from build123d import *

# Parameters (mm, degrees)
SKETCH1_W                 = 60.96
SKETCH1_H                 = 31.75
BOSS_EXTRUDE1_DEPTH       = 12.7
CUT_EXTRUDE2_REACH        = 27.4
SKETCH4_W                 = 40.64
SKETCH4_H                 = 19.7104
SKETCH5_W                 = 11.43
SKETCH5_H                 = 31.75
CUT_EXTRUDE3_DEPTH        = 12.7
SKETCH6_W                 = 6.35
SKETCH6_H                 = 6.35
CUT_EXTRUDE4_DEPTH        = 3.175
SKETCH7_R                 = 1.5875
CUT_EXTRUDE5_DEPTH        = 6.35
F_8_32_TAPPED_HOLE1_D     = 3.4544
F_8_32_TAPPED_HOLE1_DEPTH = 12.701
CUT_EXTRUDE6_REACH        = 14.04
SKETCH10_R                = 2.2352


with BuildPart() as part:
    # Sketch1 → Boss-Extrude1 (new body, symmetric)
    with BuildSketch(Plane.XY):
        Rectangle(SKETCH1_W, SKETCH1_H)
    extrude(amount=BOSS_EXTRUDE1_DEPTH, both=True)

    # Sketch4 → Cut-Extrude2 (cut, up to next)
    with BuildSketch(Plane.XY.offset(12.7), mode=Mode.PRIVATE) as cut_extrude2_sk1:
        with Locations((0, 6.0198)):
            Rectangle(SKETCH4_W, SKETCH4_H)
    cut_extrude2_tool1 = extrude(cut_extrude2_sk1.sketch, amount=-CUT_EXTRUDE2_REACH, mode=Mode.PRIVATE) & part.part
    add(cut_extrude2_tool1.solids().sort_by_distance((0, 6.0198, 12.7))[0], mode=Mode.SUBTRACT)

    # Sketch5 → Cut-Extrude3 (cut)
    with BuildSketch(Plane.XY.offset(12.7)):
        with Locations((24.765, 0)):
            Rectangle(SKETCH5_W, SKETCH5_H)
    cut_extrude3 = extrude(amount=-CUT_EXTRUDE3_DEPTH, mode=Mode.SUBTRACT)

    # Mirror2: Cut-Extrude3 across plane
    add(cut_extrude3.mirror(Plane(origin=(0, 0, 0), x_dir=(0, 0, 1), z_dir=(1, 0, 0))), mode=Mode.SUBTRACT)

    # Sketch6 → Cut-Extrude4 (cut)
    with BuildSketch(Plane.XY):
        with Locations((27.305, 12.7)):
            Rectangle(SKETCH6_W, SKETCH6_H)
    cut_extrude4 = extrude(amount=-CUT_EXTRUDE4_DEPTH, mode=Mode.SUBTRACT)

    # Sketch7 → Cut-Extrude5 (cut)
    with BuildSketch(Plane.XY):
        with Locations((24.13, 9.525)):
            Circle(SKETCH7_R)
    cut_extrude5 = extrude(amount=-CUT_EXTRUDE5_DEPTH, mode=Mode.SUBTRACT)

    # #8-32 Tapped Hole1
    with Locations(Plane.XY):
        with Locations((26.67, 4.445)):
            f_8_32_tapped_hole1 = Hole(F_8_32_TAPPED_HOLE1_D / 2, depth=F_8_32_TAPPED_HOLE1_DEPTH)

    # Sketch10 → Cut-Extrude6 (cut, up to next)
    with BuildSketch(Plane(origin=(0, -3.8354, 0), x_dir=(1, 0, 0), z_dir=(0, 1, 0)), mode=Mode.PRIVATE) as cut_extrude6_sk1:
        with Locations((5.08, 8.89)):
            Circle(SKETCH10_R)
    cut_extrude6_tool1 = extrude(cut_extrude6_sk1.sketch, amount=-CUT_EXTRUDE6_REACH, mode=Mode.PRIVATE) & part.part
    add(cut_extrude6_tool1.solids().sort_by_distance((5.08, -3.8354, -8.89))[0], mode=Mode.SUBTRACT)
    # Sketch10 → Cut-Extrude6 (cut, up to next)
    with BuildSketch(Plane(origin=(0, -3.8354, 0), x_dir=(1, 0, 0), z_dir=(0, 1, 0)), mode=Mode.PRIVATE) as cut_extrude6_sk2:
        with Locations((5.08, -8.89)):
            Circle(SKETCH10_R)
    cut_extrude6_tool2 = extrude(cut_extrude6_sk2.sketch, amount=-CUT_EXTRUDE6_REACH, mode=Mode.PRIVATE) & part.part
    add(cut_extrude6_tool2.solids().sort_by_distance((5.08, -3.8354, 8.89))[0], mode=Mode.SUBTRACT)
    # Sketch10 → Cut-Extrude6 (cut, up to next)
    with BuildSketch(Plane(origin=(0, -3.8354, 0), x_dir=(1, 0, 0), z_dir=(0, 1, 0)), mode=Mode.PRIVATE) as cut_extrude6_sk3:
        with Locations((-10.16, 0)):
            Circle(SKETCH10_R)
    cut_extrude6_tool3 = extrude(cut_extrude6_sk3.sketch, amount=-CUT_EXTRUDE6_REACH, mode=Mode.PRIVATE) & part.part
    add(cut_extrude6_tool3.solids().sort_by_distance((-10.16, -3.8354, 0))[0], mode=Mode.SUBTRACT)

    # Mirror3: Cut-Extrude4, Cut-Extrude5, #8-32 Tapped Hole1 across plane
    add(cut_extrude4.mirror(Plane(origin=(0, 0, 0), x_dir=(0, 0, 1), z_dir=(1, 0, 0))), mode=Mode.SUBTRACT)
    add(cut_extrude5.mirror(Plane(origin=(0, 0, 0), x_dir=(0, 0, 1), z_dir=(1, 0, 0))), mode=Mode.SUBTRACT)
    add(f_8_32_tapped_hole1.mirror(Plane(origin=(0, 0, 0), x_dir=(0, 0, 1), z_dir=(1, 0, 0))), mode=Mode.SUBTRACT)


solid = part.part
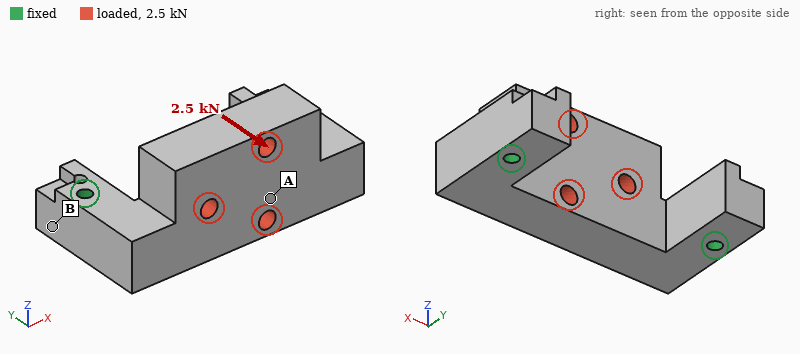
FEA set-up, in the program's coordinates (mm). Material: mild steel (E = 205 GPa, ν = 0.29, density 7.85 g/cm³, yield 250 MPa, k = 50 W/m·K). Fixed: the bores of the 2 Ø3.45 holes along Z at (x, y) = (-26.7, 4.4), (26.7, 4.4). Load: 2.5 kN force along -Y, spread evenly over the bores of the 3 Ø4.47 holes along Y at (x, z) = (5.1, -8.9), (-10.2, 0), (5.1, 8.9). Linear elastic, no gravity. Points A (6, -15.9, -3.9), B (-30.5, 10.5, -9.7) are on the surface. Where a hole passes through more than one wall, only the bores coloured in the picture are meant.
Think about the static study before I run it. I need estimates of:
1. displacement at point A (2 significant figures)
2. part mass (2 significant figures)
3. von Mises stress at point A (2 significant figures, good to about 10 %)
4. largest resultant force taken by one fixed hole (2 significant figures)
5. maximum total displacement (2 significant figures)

8.8 µm
150 g
32 MPa
1.6 kN
18 µm
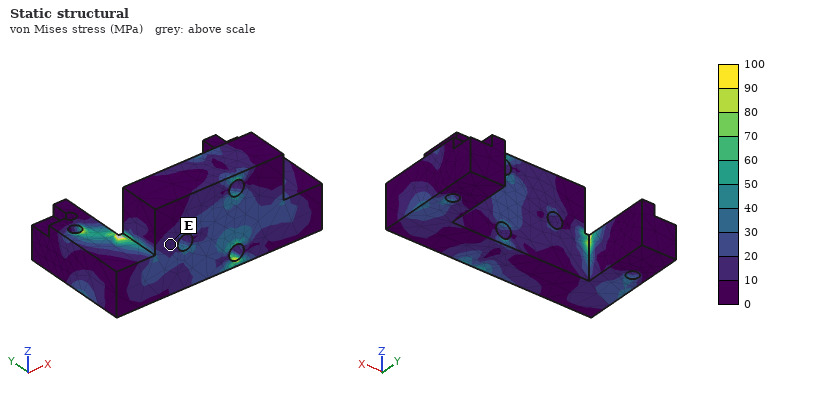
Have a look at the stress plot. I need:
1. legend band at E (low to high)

10 to 20 MPa
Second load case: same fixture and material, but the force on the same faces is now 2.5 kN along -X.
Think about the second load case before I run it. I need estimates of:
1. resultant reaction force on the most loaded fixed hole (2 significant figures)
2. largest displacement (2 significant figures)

1.4 kN
6.0 µm
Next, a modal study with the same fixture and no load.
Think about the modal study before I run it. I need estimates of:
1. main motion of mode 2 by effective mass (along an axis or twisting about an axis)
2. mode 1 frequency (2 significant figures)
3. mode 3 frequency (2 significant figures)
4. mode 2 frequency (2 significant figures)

along X
6900 Hz
12 kHz
11 kHz
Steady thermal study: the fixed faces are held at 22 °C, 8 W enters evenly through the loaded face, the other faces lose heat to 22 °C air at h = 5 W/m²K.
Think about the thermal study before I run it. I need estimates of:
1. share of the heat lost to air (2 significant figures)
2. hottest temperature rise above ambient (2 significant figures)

3.1 %
15 K
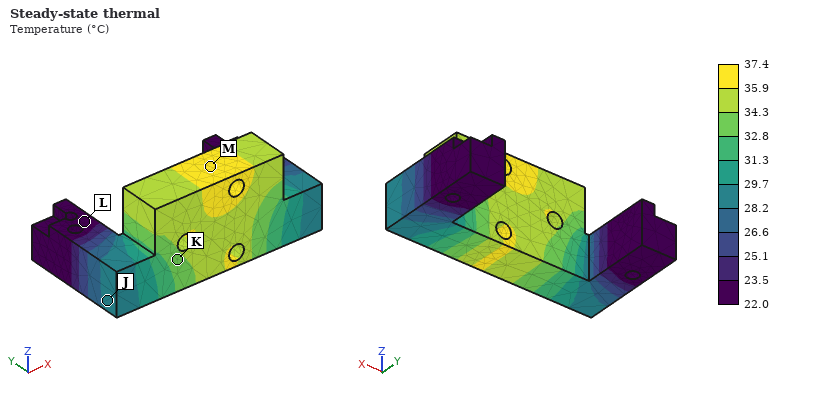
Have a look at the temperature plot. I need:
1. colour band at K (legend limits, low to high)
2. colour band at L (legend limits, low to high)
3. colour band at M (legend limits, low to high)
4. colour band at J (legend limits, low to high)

32.8 to 34.3 °C
22.0 to 23.5 °C
35.9 to 37.4 °C
28.2 to 29.7 °C
